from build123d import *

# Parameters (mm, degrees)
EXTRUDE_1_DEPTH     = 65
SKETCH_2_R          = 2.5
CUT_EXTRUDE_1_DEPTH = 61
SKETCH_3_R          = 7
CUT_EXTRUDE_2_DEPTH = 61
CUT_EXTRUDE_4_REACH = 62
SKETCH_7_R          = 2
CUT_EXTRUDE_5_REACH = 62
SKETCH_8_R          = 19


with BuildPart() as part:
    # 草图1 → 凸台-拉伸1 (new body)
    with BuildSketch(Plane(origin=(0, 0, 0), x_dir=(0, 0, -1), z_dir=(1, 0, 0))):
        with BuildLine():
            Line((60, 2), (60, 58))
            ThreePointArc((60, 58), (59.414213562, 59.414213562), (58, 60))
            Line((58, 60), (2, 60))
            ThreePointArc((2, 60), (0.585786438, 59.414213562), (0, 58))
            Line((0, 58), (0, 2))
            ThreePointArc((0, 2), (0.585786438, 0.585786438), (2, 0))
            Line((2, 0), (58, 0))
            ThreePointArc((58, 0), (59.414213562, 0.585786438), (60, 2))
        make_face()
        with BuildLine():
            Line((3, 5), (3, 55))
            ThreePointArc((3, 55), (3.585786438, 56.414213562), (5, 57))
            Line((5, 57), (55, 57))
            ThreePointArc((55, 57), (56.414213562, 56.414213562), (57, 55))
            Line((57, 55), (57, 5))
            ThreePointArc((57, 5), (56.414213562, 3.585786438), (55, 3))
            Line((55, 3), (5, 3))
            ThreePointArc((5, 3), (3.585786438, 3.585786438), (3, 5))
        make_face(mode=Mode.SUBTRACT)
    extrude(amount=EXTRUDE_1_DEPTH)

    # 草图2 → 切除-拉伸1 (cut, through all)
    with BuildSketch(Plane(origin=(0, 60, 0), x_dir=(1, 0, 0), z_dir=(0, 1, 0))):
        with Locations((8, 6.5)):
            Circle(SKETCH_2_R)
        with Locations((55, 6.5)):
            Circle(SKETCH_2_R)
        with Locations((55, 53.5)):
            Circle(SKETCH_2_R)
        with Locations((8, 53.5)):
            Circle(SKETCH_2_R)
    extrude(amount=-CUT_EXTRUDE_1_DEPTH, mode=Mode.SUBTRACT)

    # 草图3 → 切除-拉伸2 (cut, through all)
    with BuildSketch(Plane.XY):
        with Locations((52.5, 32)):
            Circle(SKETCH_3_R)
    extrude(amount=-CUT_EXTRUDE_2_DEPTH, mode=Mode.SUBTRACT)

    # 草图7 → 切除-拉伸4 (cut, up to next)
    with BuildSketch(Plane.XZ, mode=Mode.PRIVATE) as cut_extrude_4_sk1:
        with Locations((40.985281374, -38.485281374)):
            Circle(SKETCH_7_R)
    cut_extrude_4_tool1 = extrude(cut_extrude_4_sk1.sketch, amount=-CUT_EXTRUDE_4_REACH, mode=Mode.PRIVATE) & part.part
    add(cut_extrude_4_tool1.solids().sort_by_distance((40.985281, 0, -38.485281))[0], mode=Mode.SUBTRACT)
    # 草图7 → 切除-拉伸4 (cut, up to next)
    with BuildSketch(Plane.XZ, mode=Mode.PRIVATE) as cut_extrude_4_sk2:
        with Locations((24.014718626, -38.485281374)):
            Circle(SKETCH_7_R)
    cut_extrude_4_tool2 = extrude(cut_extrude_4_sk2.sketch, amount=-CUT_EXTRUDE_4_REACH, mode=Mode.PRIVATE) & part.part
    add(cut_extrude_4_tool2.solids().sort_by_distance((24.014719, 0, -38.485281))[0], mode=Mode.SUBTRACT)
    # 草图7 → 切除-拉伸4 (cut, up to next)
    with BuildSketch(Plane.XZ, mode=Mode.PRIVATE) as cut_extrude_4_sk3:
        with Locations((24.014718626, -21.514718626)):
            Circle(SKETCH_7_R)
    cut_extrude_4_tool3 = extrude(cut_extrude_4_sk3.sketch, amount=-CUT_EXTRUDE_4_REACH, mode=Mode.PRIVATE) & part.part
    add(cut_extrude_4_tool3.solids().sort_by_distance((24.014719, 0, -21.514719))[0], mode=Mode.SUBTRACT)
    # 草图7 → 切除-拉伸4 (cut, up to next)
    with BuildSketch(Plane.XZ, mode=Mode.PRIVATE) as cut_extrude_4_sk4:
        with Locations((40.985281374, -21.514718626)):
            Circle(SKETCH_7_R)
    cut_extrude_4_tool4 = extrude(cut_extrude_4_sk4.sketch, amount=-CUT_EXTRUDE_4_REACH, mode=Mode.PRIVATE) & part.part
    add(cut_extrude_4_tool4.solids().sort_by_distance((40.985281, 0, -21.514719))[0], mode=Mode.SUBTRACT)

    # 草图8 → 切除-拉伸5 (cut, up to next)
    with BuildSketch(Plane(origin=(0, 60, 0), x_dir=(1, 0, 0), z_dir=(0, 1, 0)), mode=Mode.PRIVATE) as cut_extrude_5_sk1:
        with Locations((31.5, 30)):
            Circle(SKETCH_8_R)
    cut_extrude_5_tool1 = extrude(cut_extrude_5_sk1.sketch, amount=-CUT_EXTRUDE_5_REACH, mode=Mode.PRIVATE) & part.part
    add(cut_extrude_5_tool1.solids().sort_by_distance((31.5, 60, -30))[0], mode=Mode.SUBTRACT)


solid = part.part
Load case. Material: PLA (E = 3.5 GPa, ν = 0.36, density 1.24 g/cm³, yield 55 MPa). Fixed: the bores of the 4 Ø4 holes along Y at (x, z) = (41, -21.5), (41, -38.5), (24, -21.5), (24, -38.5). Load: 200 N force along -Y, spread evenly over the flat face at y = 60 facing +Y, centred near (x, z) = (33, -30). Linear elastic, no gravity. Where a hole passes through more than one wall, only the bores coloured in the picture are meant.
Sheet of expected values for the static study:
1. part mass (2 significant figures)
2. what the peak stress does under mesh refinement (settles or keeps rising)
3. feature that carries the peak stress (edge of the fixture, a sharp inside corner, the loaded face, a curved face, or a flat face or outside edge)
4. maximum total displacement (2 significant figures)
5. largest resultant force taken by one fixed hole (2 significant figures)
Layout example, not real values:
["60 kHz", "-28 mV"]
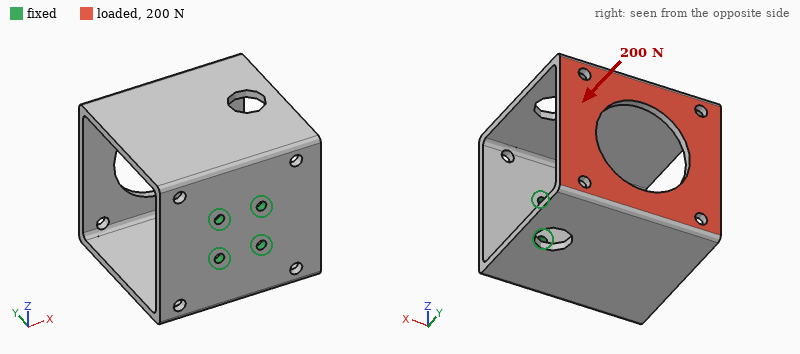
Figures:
["49 g", "keeps rising", "edge of the fixture", "1.2 mm", "52 N"]
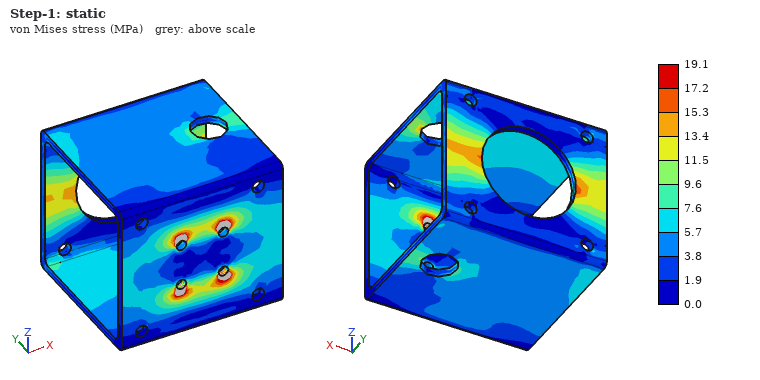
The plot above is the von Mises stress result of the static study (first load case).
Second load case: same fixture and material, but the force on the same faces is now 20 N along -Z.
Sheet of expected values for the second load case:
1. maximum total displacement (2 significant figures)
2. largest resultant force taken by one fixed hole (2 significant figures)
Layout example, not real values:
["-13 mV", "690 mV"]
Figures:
["1.1 mm", "17 N"]
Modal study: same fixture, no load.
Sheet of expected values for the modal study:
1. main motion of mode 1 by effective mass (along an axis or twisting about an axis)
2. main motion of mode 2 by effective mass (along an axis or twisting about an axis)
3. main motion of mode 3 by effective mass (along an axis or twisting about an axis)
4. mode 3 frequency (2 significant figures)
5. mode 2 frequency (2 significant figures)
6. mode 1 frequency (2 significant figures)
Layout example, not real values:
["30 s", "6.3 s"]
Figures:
["along Z", "along X", "twisting about Y", "400 Hz", "250 Hz", "160 Hz"]
